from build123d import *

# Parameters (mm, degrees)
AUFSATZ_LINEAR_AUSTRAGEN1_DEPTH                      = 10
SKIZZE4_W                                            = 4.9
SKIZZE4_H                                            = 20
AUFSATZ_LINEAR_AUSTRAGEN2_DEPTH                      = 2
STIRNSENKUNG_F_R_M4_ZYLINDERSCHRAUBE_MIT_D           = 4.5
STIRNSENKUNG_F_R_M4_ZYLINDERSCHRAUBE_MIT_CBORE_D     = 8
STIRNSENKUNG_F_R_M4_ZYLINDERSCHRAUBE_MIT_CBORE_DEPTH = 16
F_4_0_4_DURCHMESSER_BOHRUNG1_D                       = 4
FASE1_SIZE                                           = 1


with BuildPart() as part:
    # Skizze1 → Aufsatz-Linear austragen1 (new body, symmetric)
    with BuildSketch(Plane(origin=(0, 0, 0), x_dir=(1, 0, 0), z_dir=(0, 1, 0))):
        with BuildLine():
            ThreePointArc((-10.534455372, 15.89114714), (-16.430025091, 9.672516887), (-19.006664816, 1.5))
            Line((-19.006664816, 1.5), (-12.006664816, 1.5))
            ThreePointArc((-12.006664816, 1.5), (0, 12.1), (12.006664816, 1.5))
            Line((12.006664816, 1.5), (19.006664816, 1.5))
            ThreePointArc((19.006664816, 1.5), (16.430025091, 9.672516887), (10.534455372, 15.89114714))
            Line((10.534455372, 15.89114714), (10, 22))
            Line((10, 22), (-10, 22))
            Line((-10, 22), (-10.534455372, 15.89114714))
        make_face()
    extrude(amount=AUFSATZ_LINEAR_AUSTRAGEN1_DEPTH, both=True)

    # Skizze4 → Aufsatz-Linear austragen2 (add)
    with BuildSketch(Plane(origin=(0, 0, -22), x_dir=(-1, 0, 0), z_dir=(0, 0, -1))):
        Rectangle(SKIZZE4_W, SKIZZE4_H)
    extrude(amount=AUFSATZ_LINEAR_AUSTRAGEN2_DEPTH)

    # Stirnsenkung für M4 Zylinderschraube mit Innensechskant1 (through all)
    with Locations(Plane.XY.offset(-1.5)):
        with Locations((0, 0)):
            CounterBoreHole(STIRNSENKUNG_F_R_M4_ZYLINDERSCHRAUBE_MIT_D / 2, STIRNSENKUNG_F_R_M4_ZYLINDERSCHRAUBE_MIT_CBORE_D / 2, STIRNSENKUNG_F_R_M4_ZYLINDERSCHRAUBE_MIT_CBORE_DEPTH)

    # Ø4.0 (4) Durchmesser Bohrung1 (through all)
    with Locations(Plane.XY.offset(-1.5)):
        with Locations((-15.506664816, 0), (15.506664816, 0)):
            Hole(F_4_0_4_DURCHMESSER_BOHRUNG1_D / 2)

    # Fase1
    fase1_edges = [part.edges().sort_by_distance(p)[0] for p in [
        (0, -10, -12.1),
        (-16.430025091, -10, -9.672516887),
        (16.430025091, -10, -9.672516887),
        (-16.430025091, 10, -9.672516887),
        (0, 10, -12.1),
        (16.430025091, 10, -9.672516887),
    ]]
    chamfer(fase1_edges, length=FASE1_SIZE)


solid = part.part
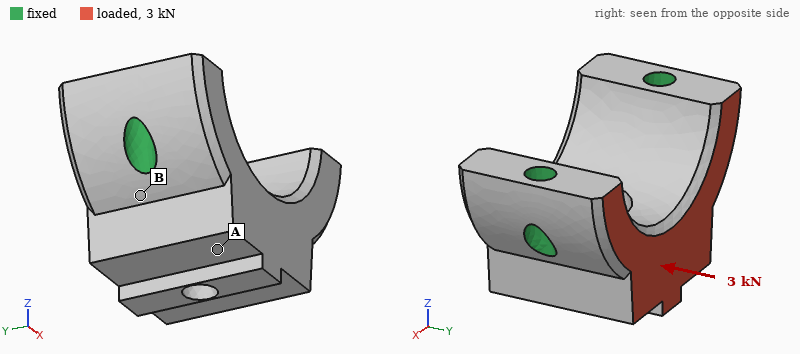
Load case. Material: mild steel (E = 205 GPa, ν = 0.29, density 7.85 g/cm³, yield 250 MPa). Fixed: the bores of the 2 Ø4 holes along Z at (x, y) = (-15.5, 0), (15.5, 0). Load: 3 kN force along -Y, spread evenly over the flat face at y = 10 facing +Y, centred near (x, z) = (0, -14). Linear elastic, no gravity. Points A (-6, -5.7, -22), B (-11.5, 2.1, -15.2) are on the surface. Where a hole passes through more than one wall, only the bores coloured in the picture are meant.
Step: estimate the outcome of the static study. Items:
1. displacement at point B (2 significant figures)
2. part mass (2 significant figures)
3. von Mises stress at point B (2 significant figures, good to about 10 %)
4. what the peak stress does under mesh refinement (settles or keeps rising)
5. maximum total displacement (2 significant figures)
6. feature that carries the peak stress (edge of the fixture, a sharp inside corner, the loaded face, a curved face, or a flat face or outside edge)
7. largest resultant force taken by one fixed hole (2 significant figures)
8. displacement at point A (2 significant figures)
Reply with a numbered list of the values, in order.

1. 2.1 µm
2. 59 g
3. 37 MPa
4. keeps rising
5. 6.5 µm
6. edge of the fixture
7. 1.5 kN
8. 4.6 µm
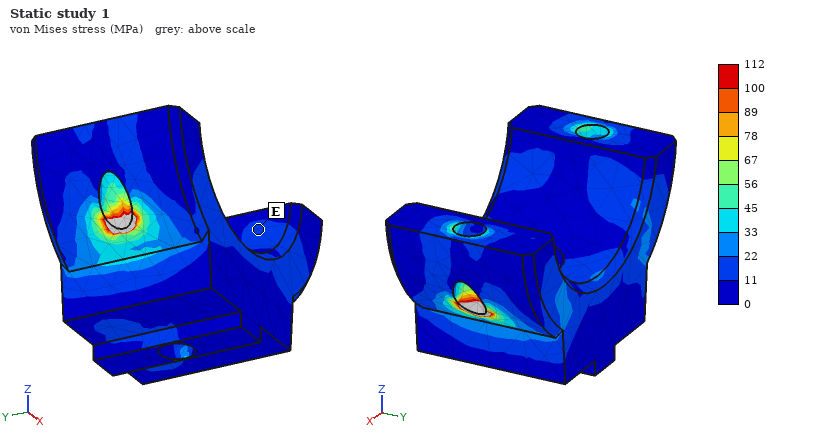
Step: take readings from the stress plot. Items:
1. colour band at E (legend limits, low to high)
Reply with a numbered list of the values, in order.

1. 11 to 22 MPa
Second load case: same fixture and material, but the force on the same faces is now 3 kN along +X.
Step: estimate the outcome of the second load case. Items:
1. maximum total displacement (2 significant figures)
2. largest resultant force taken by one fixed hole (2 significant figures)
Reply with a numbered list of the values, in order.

1. 3.4 µm
2. 1.8 kN
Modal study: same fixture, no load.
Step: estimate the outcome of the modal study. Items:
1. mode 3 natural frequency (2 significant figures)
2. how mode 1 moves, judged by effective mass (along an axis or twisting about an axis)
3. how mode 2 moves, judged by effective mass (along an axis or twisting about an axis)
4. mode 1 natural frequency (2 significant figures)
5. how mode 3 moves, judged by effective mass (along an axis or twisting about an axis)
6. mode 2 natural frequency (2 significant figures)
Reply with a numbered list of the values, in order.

1. 38 kHz
2. along Y
3. along Z
4. 18 kHz
5. along X
6. 35 kHz
